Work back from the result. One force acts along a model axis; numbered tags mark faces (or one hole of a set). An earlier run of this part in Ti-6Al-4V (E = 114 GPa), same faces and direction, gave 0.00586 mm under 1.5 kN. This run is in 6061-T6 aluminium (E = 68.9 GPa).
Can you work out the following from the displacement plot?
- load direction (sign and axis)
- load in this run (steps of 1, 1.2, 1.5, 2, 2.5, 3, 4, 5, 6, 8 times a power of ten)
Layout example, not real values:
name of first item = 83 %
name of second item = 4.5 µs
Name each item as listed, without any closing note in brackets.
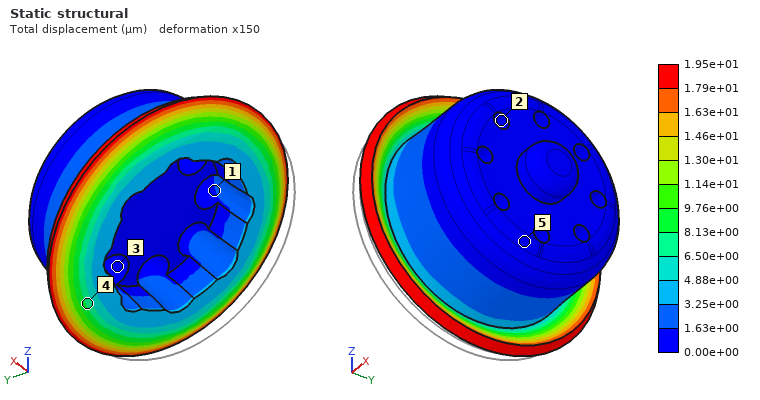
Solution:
load direction = +X
load in this run = 3 kN
